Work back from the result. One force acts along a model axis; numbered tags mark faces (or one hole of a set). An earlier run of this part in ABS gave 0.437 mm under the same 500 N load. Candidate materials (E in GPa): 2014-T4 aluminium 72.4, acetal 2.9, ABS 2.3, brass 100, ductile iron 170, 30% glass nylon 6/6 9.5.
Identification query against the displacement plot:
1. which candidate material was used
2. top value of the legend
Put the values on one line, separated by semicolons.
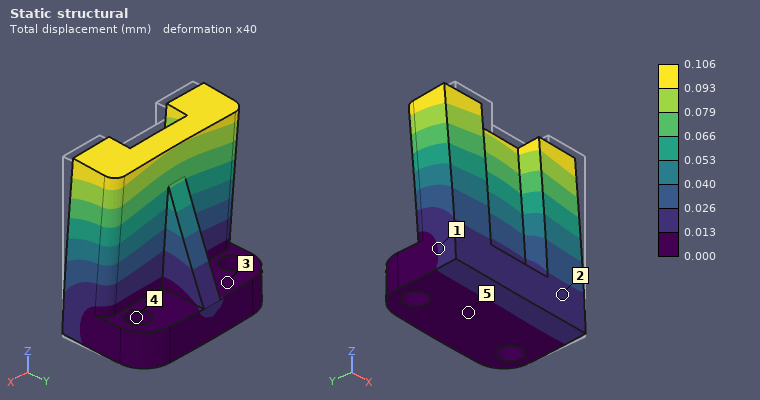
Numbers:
30% glass nylon 6/6; 0.106 mm
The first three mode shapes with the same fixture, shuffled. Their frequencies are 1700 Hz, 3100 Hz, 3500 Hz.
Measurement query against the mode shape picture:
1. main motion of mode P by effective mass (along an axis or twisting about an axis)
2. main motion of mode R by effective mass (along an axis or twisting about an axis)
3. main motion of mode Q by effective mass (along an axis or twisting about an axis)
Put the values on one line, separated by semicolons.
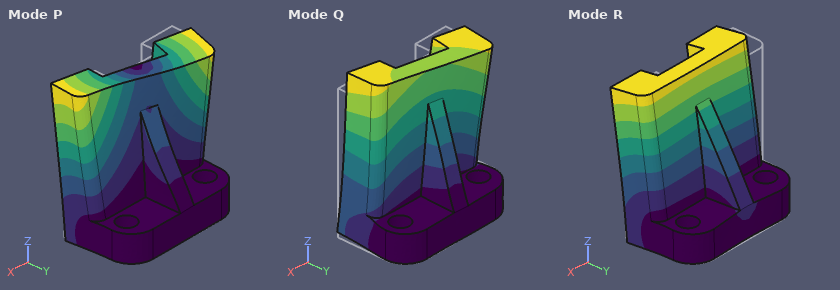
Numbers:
twisting about Z; along Y; along X
